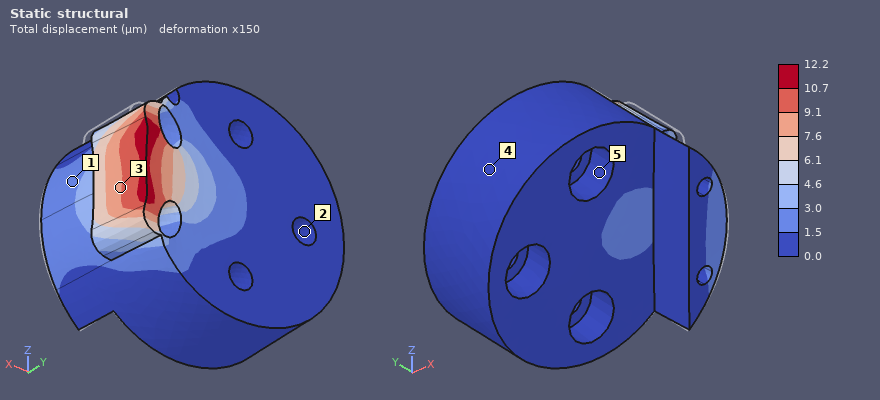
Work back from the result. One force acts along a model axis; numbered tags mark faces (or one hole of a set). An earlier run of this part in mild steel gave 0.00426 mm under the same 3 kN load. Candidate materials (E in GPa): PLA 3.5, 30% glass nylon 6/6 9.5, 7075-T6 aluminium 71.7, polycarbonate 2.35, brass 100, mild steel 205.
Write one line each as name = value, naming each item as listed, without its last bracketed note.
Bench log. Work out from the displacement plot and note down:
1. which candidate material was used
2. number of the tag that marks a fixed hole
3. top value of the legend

which candidate material was used = 7075-T6 aluminium
number of the tag that marks a fixed hole = 2
top value of the legend = 12.2 µm
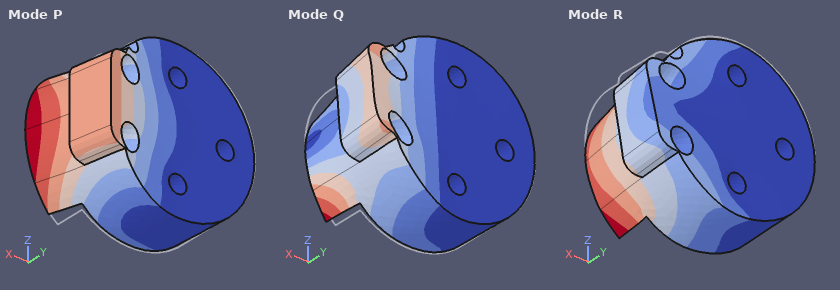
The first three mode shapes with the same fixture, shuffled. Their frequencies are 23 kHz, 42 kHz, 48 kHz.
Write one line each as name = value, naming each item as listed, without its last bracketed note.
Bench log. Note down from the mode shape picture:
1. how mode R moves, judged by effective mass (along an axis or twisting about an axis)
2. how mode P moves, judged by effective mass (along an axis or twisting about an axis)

how mode R moves, judged by effective mass = along Z
how mode P moves, judged by effective mass = along Y
